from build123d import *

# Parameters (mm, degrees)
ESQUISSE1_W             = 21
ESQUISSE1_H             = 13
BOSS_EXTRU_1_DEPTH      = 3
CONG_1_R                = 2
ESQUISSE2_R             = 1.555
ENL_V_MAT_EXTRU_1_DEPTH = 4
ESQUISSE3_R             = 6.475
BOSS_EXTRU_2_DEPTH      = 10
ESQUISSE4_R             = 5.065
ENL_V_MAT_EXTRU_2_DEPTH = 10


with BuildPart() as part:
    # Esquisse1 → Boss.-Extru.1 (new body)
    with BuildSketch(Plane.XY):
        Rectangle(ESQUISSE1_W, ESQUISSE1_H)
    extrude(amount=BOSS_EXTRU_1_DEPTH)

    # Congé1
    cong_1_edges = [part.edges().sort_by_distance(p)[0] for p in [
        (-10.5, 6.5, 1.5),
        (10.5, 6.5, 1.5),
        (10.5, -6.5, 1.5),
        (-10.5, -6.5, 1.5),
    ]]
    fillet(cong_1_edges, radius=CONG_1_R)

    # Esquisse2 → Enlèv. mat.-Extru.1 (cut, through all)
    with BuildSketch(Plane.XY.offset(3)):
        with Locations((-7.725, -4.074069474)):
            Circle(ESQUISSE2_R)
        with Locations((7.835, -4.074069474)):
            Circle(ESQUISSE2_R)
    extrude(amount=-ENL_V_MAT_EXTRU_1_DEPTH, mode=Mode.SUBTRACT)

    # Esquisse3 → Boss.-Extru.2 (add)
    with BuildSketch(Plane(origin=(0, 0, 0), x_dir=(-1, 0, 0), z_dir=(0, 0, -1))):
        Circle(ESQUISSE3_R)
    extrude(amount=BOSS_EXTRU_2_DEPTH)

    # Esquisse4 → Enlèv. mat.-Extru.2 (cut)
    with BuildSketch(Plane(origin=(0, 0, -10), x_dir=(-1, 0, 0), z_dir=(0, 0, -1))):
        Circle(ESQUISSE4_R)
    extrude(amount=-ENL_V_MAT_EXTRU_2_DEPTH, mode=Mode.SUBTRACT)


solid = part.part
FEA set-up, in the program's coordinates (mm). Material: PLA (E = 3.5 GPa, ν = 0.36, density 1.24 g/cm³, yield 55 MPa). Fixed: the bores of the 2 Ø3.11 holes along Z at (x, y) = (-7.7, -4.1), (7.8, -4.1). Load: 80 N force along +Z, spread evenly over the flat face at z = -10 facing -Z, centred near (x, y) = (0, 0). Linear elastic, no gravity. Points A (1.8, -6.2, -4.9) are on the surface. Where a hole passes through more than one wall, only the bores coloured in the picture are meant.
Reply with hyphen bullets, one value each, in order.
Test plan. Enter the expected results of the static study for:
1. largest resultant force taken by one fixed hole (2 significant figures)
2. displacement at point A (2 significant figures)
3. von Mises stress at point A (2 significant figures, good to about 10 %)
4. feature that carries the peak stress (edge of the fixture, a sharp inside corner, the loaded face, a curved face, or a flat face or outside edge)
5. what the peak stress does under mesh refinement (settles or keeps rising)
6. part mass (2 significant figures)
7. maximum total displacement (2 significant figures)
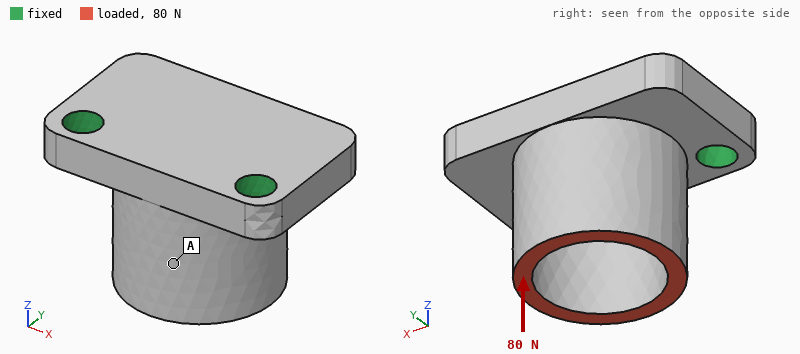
- 41 N
- 21 µm
- 1.7 MPa
- edge of the fixture
- keeps rising
- 1.6 g
- 88 µm
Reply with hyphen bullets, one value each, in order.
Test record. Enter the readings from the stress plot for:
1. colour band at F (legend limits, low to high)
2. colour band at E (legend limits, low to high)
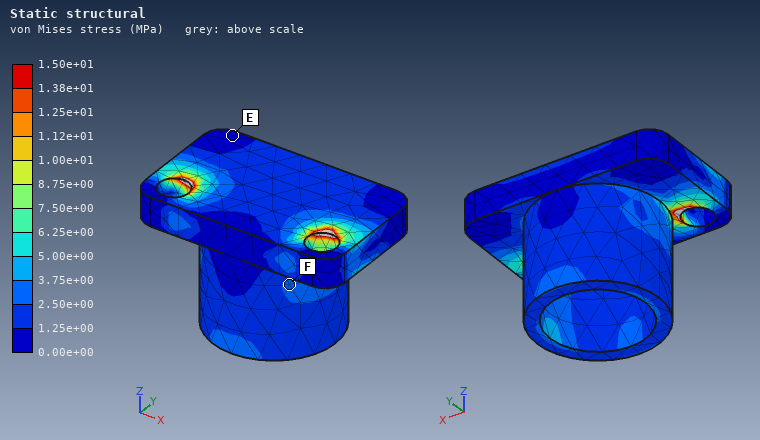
- 2.50e+00 to 3.75e+00 MPa
- 0.00e+00 to 1.25e+00 MPa
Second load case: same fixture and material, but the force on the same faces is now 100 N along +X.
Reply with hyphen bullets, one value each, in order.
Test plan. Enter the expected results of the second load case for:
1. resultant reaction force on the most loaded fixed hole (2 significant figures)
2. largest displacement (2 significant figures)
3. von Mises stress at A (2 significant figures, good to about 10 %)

- 100 N
- 0.10 mm
- 7.9 MPa
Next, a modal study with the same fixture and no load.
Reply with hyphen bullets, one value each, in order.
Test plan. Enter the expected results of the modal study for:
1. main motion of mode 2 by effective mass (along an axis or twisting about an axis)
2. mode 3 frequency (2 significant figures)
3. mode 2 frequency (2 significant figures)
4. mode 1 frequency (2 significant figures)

- along X
- 11 kHz
- 9300 Hz
- 4400 Hz
